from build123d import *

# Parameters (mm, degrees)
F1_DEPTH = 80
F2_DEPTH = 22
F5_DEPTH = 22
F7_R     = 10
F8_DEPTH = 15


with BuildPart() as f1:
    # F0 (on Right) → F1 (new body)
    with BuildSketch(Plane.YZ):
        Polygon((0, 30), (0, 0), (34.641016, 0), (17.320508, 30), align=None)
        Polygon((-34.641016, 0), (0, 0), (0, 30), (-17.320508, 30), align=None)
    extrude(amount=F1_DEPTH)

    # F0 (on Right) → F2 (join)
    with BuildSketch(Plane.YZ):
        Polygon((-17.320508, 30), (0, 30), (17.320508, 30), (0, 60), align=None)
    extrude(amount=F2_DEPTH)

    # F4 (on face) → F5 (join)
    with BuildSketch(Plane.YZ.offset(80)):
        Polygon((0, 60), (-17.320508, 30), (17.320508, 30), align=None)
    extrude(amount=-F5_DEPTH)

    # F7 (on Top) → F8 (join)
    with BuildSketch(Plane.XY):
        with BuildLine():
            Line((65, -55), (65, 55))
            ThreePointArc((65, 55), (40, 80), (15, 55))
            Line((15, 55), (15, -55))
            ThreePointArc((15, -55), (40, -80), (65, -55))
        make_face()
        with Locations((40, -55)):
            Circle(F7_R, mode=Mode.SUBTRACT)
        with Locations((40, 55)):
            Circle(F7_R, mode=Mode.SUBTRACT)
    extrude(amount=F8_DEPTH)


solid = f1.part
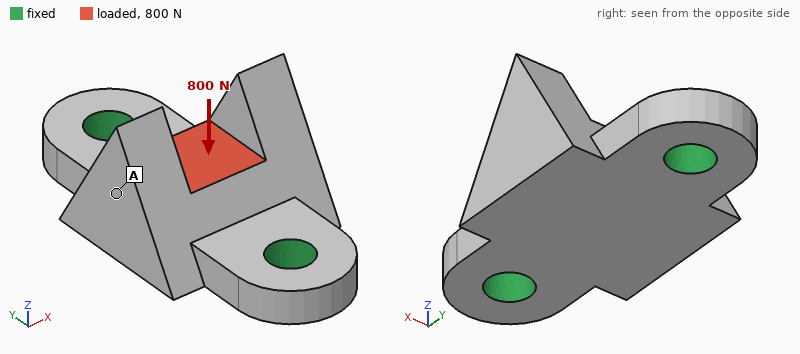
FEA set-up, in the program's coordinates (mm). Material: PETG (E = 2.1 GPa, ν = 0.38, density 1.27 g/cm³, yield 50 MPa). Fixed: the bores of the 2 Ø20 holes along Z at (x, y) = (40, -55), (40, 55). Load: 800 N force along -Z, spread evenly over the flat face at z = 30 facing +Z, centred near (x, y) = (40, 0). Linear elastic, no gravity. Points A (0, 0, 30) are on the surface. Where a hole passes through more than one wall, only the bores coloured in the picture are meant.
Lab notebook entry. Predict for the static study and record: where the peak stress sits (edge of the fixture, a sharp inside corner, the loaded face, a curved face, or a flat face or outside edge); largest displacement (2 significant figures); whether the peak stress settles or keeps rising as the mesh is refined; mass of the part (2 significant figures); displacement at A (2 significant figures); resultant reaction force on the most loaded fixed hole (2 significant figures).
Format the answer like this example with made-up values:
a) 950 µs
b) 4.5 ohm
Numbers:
a) edge of the fixture
b) 64 µm
c) keeps rising
d) 260 g
e) 61 µm
f) 430 N
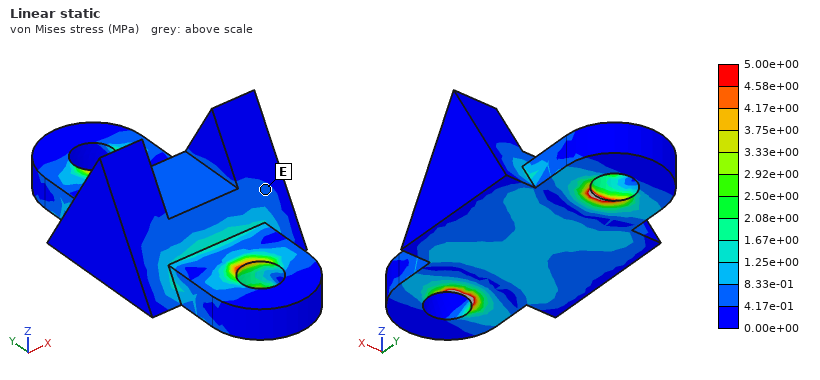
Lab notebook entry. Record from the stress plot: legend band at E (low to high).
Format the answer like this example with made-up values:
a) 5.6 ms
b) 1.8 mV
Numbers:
a) 4.17e-01 to 8.33e-01 MPa
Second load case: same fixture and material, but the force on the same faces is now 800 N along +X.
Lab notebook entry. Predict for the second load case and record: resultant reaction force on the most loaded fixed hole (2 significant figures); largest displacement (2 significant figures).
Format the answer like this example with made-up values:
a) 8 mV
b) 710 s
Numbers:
a) 400 N
b) 0.35 mm
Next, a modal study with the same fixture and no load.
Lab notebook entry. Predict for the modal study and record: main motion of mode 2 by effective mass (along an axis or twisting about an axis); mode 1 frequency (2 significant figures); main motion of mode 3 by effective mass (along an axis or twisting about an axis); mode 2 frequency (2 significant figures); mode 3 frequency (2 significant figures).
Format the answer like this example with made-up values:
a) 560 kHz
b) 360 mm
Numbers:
a) along Z
b) 760 Hz
c) along X
d) 1300 Hz
e) 2100 Hz
